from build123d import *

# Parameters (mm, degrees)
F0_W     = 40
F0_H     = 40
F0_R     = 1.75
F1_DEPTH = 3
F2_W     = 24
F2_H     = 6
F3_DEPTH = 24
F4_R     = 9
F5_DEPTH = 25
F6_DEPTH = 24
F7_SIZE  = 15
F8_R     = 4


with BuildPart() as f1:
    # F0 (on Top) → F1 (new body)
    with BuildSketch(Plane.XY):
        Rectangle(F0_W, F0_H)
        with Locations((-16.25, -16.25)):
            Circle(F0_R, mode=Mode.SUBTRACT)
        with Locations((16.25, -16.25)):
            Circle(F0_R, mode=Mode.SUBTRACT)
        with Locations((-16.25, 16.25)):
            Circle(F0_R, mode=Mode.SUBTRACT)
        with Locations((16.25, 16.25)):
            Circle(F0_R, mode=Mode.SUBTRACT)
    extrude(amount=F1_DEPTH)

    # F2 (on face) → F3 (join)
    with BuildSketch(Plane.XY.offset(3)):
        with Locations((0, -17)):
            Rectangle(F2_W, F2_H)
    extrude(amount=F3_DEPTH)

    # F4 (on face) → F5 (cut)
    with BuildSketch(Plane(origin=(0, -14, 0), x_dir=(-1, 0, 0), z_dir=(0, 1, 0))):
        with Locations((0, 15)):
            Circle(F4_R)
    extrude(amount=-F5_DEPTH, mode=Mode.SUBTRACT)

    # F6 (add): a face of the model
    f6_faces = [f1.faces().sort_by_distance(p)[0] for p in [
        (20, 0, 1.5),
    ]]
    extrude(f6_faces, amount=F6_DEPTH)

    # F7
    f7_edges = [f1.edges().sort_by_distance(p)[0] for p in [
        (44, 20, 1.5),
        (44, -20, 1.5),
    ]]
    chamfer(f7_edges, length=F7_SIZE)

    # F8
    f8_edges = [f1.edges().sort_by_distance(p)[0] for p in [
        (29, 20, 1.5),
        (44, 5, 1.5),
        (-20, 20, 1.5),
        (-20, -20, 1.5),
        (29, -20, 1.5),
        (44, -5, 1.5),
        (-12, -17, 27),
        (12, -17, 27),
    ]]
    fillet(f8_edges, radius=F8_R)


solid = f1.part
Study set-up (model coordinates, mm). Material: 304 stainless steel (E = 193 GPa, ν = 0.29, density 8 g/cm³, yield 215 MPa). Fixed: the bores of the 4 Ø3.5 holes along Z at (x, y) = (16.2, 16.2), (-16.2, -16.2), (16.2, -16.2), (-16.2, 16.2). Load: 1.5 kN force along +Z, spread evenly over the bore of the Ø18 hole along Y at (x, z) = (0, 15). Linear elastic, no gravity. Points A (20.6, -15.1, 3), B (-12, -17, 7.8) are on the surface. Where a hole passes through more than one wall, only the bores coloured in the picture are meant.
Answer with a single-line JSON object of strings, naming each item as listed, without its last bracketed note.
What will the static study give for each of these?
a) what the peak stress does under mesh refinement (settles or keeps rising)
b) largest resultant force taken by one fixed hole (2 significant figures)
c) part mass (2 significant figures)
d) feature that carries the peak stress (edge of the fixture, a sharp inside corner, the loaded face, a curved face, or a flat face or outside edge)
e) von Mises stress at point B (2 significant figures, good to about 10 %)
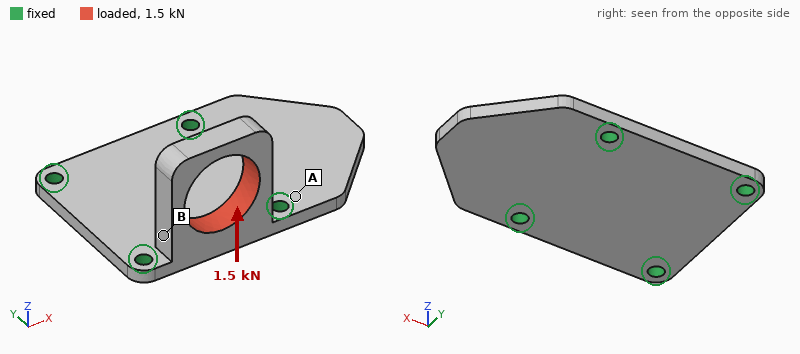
{"what the peak stress does under mesh refinement": "keeps rising", "largest resultant force taken by one fixed hole": "820 N", "part mass": "70 g", "feature that carries the peak stress": "edge of the fixture", "von Mises stress at point B": "49 MPa"}
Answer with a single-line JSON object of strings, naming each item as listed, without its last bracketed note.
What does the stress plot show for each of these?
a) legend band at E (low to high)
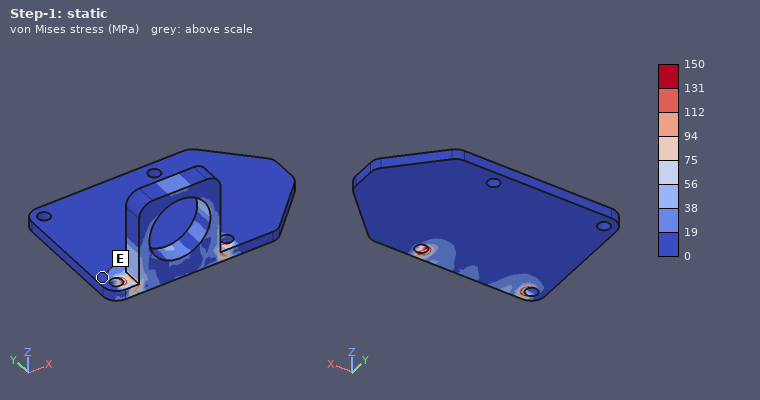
{"legend band at E": "0 to 19 MPa"}
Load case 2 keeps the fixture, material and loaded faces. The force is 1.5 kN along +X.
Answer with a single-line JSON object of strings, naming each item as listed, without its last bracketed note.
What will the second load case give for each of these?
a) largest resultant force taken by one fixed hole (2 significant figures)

{"largest resultant force taken by one fixed hole": "1.0 kN"}
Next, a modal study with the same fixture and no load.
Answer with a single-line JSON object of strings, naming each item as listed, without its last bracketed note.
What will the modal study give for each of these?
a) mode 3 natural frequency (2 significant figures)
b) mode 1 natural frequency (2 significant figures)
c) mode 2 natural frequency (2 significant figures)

{"mode 3 natural frequency": "8900 Hz", "mode 1 natural frequency": "3700 Hz", "mode 2 natural frequency": "4000 Hz"}
